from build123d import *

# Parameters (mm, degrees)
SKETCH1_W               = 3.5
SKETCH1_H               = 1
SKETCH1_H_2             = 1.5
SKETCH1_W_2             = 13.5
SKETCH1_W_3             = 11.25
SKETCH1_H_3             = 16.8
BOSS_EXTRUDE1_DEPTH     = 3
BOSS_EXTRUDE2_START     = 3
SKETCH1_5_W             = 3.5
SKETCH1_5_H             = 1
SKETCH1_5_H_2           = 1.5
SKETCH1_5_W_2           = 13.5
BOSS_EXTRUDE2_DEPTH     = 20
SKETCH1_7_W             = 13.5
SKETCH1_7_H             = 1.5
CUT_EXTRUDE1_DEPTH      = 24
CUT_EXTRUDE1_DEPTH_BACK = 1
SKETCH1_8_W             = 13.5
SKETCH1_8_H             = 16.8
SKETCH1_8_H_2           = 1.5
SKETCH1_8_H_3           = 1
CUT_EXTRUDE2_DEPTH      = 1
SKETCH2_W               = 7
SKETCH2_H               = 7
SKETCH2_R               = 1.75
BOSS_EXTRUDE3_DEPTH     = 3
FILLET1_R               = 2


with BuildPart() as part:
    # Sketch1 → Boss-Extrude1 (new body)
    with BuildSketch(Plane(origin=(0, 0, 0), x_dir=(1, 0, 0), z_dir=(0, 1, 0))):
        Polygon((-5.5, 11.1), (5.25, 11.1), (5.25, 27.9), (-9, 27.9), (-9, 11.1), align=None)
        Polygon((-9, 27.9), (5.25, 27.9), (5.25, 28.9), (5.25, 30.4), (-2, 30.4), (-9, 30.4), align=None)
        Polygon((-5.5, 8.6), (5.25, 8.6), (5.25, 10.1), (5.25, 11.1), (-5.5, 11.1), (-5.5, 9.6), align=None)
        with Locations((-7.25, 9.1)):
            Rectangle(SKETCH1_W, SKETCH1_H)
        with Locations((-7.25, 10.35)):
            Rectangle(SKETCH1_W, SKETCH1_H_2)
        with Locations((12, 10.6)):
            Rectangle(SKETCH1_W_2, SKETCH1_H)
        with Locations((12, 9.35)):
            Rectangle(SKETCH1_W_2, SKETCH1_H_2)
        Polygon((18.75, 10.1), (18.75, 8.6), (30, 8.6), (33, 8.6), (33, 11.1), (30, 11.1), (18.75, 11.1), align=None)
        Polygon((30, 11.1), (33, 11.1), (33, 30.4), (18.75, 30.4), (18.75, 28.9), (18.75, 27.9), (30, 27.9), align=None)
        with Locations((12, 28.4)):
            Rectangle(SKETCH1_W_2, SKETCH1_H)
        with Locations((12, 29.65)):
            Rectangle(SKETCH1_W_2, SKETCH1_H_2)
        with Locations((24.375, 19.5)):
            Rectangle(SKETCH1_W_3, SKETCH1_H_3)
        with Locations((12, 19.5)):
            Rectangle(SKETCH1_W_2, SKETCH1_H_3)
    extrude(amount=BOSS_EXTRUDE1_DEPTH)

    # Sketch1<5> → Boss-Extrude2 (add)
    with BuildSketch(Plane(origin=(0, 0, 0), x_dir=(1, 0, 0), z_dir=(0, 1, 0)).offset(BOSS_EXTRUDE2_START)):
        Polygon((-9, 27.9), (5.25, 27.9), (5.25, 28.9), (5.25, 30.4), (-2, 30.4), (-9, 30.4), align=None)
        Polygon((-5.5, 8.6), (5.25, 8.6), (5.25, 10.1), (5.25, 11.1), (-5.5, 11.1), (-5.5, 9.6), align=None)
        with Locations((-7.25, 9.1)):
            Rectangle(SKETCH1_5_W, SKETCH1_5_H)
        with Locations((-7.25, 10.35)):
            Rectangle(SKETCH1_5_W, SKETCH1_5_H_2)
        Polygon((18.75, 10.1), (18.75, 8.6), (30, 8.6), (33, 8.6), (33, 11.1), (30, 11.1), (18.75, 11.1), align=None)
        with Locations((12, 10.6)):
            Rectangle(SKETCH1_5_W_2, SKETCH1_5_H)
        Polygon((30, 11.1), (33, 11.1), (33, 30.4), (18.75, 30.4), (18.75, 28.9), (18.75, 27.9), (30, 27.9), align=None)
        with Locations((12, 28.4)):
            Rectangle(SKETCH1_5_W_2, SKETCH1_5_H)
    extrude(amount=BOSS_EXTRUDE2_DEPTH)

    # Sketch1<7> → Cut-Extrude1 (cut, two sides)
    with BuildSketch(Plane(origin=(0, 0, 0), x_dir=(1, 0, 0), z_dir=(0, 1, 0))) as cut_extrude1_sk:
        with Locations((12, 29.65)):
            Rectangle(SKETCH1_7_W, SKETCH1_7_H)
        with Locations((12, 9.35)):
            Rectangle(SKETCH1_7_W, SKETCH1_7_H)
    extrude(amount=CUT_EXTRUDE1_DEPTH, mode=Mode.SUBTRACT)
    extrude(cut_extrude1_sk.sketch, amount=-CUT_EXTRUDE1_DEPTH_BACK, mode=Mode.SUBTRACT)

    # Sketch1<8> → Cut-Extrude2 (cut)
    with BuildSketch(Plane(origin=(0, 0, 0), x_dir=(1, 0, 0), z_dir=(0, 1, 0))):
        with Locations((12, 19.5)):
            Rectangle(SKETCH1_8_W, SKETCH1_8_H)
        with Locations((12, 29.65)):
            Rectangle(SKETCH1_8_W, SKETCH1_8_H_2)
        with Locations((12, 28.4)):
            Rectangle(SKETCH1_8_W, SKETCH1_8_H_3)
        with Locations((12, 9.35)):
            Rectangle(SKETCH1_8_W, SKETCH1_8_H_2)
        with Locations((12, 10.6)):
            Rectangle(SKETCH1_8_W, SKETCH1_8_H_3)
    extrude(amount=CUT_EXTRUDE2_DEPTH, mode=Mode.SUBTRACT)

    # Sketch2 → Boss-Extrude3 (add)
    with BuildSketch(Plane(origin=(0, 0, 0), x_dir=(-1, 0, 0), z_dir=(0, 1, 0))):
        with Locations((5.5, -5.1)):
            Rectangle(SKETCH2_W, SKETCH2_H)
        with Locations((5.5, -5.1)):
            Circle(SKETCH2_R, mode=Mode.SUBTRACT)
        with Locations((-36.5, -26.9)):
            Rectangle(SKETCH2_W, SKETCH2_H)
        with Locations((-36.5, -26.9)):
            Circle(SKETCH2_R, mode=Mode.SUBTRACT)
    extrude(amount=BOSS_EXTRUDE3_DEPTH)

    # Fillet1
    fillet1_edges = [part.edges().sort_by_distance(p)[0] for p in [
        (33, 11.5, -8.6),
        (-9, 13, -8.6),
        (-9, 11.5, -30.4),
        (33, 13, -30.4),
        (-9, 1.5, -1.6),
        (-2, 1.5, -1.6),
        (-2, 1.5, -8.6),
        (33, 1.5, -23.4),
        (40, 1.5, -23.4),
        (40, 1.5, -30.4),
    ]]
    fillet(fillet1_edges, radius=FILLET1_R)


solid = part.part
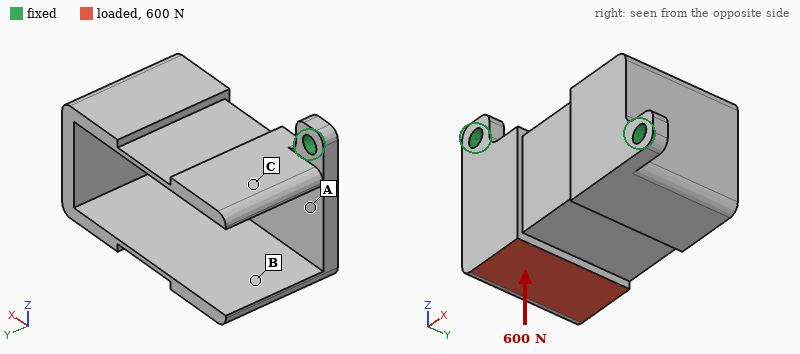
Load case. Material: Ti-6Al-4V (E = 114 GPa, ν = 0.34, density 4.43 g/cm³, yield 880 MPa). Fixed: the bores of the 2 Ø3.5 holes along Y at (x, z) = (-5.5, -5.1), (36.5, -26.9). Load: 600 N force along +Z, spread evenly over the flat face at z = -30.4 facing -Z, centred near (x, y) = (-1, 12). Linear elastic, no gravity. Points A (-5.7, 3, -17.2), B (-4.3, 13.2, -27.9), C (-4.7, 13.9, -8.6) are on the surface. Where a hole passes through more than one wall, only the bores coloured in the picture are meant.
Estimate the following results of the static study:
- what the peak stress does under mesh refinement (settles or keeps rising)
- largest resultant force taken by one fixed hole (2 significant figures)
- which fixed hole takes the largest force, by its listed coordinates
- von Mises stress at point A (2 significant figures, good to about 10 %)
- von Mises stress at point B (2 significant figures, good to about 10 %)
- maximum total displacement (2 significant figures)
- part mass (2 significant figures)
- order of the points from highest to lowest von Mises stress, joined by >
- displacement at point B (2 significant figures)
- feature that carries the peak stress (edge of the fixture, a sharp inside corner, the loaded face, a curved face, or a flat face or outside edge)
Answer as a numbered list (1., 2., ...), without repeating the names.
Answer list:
1. keeps rising
2. 530 N
3. (-5.5, -5.1)
4. 130 MPa
5. 76 MPa
6. 0.59 mm
7. 31 g
8. A > B > C
9. 0.30 mm
10. edge of the fixture
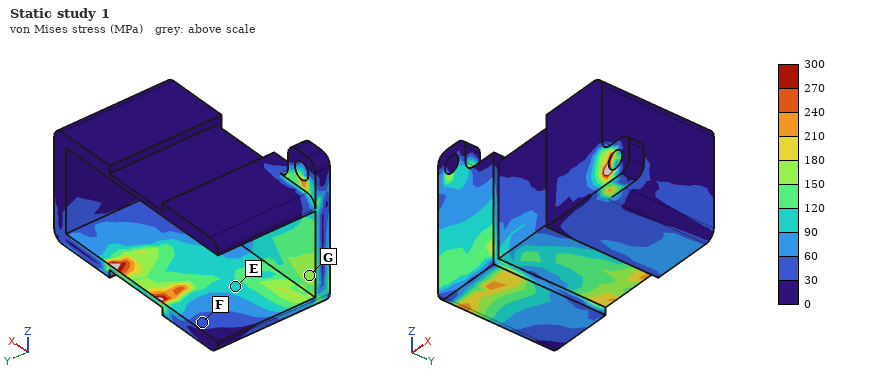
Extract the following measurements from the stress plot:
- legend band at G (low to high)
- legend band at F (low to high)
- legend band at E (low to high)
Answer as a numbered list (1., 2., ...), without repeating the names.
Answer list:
1. 150 to 180 MPa
2. 30 to 60 MPa
3. 90 to 120 MPa
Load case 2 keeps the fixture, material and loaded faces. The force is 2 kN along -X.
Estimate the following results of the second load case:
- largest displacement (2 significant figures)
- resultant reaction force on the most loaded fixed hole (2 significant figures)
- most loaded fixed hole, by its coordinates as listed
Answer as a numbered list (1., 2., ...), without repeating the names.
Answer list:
1. 0.37 mm
2. 1.7 kN
3. (36.5, -26.9)
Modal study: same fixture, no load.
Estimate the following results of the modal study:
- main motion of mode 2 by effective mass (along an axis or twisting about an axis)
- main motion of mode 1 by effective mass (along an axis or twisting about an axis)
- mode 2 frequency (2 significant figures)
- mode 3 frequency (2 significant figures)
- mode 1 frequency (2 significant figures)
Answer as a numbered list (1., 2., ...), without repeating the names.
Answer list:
1. along Y
2. along Z
3. 3600 Hz
4. 4100 Hz
5. 2100 Hz
